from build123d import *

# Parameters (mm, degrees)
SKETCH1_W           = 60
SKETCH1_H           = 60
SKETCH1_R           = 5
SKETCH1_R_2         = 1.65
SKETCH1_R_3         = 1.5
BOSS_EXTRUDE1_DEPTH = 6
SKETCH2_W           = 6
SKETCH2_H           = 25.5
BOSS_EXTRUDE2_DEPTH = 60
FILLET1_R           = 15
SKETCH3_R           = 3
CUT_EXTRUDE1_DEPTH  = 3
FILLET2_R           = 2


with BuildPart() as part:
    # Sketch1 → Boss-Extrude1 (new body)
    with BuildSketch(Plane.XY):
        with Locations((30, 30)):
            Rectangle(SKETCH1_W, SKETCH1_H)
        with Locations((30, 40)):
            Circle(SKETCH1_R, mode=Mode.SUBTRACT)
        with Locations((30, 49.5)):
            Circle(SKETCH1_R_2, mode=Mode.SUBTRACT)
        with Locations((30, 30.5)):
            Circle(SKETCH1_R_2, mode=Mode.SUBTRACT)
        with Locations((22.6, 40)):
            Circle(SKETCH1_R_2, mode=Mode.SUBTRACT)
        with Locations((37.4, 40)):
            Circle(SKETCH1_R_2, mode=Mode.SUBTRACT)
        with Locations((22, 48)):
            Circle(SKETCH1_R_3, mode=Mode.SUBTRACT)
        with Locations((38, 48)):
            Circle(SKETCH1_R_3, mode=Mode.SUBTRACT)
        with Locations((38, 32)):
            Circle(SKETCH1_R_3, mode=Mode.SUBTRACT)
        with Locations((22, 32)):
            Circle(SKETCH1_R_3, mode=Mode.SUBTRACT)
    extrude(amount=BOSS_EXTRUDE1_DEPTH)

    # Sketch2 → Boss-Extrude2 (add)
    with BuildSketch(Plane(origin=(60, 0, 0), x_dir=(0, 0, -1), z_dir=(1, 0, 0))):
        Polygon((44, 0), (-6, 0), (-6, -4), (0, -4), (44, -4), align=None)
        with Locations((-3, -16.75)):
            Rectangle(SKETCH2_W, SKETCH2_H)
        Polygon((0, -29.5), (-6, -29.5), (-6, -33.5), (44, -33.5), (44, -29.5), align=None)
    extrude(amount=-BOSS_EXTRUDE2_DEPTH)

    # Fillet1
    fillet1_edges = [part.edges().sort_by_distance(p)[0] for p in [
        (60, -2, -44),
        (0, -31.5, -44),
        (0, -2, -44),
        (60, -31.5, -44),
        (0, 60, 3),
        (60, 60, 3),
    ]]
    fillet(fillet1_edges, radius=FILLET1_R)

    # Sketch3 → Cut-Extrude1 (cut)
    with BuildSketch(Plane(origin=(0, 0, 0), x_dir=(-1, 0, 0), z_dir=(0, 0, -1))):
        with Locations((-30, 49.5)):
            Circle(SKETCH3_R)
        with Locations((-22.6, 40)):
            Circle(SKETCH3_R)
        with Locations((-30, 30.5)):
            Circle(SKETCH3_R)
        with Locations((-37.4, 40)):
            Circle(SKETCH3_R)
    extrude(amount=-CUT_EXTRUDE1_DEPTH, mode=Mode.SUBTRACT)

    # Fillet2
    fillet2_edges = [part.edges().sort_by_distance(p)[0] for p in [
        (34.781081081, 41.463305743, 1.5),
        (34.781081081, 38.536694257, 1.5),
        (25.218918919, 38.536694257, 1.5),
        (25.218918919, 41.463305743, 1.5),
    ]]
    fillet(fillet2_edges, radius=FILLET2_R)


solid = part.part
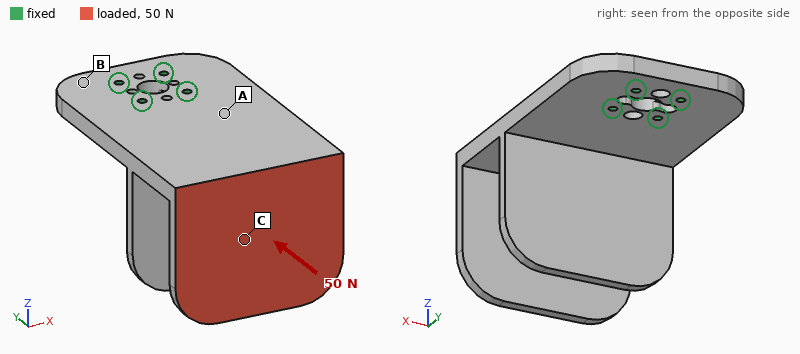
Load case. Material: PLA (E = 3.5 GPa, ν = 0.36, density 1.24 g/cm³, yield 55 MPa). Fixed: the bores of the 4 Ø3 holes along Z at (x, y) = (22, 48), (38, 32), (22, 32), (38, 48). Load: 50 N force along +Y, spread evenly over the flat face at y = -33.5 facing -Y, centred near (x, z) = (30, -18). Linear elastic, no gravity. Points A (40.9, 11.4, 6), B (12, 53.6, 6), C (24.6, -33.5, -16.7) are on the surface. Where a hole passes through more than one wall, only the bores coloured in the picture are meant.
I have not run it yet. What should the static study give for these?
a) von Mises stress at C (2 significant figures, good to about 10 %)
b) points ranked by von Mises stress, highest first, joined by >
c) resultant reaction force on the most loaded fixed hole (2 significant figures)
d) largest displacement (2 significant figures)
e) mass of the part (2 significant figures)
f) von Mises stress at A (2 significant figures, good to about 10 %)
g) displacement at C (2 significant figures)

1.9 MPa
A > C > B
25 N
1.4 mm
65 g
2.5 MPa
0.76 mm
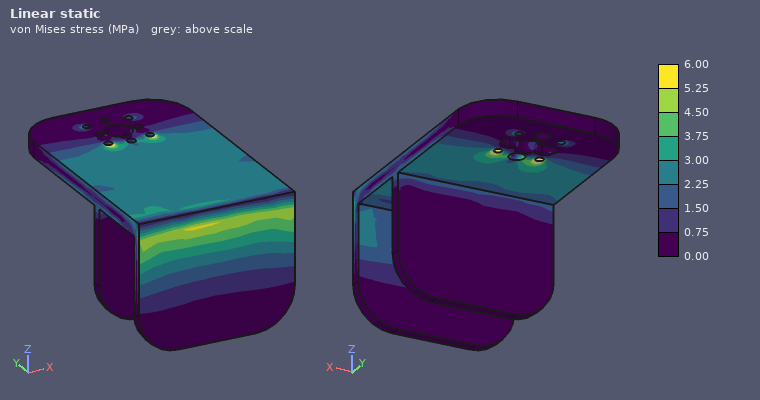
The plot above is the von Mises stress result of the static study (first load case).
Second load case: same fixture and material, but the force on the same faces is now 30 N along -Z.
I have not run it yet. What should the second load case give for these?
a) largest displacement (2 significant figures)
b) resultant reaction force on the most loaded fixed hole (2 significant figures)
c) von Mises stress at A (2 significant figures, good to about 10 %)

1.2 mm
39 N
3.3 MPa
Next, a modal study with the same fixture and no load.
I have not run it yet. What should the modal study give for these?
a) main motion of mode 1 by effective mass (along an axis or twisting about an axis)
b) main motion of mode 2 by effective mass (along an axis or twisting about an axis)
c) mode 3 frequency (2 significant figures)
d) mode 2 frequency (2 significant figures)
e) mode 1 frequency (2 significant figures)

along Z
along X
480 Hz
350 Hz
180 Hz
